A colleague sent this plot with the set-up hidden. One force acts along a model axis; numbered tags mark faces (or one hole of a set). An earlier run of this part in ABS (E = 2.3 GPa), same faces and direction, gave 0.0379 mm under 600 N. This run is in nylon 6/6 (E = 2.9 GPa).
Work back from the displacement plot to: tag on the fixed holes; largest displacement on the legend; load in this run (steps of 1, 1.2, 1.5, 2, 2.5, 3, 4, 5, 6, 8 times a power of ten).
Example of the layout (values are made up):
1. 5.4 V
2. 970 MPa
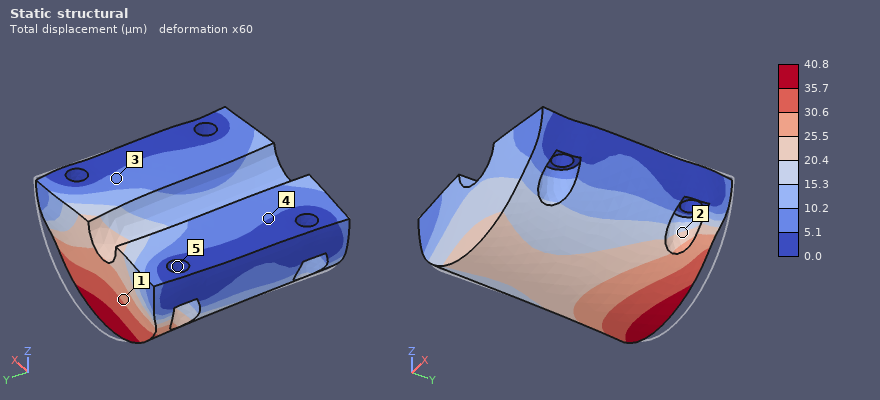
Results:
1. 5
2. 40.8 µm
3. 800 N
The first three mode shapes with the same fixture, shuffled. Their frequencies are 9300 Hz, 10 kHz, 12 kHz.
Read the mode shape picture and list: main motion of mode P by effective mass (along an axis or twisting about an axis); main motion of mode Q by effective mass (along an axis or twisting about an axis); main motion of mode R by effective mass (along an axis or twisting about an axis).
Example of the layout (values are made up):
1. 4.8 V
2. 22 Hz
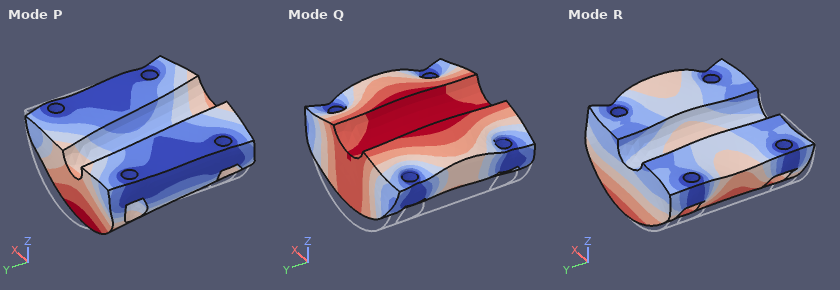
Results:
1. along Y
2. along Z
3. along X
